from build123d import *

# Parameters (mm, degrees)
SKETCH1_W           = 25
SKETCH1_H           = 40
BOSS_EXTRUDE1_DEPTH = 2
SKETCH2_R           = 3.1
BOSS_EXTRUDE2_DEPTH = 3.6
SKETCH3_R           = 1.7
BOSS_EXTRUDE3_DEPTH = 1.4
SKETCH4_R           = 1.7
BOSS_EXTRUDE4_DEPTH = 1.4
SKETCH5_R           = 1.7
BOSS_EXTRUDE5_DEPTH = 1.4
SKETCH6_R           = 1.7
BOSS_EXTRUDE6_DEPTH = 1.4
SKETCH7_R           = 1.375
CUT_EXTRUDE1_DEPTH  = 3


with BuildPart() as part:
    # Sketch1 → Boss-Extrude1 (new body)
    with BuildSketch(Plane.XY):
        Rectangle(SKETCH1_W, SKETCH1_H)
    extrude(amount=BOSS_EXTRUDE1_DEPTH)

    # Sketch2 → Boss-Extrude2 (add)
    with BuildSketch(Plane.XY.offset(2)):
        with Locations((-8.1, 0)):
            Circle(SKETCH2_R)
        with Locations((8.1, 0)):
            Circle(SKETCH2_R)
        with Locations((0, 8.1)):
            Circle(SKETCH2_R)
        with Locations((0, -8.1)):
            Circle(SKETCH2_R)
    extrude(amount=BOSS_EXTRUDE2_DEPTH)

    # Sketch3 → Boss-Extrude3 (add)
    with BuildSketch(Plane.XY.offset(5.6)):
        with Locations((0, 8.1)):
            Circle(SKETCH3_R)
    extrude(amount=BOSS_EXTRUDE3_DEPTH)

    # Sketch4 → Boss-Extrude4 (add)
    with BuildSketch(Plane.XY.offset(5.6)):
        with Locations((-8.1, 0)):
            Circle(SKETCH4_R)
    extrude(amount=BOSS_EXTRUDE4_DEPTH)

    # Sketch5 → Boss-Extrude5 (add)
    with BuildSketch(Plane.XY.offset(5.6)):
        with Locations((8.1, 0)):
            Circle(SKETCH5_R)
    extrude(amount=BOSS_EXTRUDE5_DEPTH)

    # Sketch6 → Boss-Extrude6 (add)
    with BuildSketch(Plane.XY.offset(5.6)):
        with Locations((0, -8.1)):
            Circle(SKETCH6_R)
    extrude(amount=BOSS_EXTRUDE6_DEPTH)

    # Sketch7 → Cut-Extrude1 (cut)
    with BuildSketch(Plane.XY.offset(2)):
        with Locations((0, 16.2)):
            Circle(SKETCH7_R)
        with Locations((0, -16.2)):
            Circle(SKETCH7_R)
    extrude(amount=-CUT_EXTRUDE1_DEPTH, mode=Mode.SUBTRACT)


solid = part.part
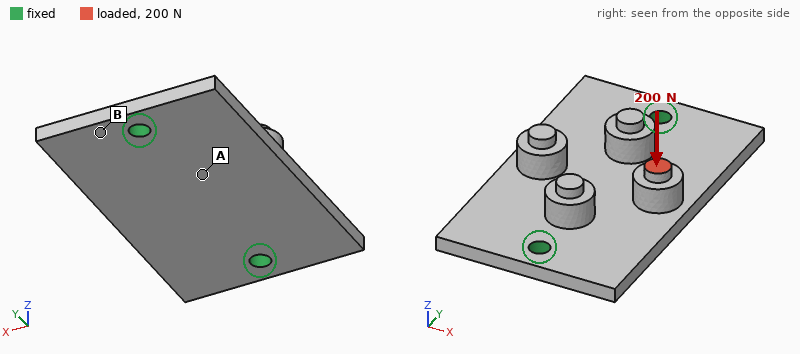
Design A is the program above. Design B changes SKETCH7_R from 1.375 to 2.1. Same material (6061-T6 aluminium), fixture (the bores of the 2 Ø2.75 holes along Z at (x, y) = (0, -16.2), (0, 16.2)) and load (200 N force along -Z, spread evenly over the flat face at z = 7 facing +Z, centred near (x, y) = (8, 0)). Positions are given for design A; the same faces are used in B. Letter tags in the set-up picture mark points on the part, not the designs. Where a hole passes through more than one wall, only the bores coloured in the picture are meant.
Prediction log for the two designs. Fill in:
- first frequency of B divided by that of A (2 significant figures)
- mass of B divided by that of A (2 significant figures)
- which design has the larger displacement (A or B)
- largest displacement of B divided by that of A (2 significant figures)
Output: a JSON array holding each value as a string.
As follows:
["1.2", "0.99", "A", "0.82"]
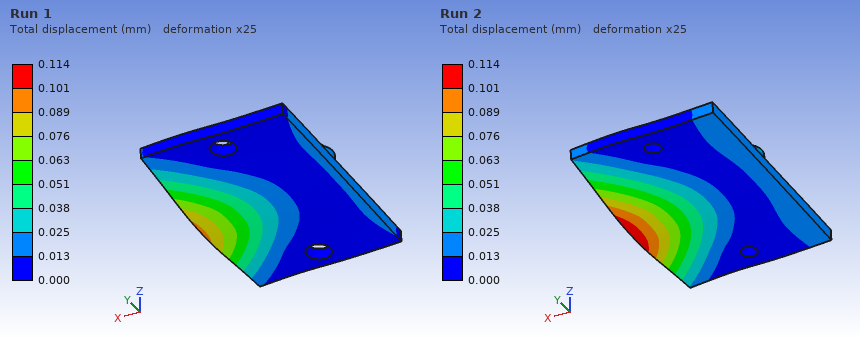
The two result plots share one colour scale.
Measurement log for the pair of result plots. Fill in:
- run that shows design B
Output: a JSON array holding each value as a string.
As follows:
["Run 1"]
